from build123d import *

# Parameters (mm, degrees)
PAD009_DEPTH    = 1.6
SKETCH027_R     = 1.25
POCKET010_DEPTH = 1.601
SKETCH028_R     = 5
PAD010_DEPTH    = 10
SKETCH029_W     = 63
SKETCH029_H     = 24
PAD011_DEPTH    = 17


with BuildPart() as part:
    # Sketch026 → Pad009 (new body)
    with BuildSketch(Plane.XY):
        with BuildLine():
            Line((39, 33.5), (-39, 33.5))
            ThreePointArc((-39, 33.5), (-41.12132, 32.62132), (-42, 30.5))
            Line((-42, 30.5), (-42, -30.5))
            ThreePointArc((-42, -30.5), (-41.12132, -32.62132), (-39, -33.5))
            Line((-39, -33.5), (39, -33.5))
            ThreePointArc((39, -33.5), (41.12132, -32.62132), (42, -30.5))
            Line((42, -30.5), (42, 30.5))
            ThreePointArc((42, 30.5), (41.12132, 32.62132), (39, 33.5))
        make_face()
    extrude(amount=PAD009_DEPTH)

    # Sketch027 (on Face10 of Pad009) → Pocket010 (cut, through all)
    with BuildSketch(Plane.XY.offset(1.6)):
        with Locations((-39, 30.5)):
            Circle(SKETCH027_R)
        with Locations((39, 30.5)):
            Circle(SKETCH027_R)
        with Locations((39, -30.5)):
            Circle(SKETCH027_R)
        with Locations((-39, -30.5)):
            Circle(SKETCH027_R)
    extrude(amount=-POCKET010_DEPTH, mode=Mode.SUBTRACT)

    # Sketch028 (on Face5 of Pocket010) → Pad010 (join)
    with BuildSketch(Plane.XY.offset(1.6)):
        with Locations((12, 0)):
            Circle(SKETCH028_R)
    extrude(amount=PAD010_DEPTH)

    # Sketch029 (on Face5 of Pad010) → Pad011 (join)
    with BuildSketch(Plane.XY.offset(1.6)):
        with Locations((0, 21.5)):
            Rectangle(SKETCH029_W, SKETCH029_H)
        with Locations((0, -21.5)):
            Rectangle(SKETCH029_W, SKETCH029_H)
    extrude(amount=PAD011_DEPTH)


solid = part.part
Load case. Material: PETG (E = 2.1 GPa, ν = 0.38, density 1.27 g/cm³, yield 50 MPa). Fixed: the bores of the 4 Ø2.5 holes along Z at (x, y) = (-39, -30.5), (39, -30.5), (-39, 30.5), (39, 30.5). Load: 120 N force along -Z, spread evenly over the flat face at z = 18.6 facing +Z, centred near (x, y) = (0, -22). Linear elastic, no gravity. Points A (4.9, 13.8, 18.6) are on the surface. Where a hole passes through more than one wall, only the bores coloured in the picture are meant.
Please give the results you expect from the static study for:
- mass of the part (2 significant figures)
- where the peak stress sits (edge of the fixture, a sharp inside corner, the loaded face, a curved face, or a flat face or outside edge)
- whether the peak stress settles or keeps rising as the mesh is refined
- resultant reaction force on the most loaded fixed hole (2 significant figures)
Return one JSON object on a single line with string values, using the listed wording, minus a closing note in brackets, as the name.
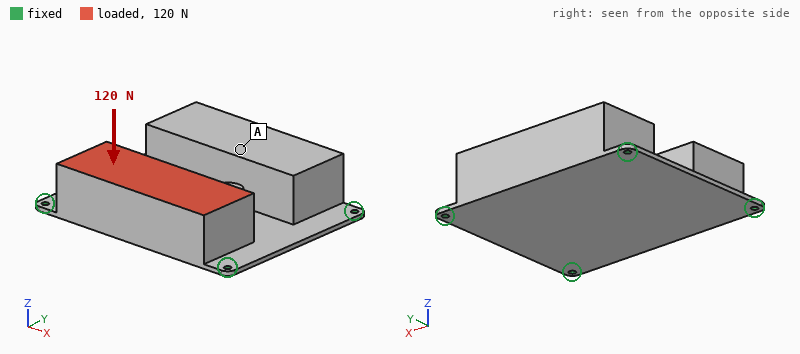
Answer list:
{"mass of the part": "78 g", "where the peak stress sits": "edge of the fixture", "whether the peak stress settles or keeps rising as the mesh is refined": "keeps rising", "resultant reaction force on the most loaded fixed hole": "60 N"}
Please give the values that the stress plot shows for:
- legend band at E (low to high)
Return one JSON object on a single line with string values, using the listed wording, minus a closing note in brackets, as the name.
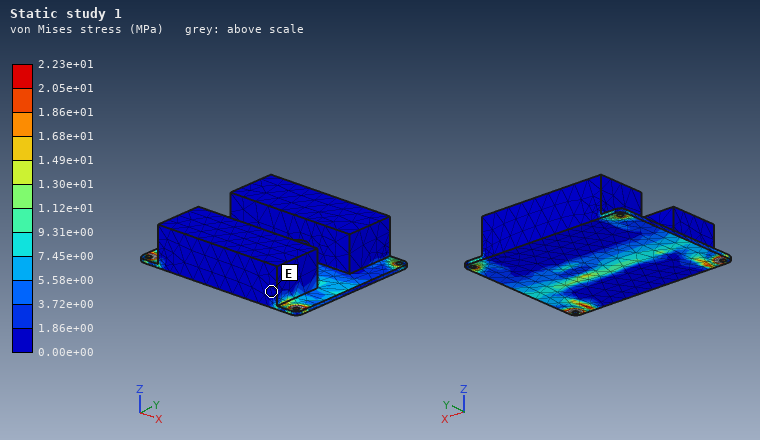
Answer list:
{"legend band at E": "0.00e+00 to 1.86e+00 MPa"}
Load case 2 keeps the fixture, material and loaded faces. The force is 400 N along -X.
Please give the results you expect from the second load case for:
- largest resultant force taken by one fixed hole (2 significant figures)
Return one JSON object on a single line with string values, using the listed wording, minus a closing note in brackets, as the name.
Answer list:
{"largest resultant force taken by one fixed hole": "180 N"}
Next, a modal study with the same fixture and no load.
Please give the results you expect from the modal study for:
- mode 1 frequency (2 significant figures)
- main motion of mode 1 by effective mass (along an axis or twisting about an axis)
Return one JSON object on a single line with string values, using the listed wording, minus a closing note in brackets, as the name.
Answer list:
{"mode 1 frequency": "180 Hz", "main motion of mode 1 by effective mass": "along Z"}
